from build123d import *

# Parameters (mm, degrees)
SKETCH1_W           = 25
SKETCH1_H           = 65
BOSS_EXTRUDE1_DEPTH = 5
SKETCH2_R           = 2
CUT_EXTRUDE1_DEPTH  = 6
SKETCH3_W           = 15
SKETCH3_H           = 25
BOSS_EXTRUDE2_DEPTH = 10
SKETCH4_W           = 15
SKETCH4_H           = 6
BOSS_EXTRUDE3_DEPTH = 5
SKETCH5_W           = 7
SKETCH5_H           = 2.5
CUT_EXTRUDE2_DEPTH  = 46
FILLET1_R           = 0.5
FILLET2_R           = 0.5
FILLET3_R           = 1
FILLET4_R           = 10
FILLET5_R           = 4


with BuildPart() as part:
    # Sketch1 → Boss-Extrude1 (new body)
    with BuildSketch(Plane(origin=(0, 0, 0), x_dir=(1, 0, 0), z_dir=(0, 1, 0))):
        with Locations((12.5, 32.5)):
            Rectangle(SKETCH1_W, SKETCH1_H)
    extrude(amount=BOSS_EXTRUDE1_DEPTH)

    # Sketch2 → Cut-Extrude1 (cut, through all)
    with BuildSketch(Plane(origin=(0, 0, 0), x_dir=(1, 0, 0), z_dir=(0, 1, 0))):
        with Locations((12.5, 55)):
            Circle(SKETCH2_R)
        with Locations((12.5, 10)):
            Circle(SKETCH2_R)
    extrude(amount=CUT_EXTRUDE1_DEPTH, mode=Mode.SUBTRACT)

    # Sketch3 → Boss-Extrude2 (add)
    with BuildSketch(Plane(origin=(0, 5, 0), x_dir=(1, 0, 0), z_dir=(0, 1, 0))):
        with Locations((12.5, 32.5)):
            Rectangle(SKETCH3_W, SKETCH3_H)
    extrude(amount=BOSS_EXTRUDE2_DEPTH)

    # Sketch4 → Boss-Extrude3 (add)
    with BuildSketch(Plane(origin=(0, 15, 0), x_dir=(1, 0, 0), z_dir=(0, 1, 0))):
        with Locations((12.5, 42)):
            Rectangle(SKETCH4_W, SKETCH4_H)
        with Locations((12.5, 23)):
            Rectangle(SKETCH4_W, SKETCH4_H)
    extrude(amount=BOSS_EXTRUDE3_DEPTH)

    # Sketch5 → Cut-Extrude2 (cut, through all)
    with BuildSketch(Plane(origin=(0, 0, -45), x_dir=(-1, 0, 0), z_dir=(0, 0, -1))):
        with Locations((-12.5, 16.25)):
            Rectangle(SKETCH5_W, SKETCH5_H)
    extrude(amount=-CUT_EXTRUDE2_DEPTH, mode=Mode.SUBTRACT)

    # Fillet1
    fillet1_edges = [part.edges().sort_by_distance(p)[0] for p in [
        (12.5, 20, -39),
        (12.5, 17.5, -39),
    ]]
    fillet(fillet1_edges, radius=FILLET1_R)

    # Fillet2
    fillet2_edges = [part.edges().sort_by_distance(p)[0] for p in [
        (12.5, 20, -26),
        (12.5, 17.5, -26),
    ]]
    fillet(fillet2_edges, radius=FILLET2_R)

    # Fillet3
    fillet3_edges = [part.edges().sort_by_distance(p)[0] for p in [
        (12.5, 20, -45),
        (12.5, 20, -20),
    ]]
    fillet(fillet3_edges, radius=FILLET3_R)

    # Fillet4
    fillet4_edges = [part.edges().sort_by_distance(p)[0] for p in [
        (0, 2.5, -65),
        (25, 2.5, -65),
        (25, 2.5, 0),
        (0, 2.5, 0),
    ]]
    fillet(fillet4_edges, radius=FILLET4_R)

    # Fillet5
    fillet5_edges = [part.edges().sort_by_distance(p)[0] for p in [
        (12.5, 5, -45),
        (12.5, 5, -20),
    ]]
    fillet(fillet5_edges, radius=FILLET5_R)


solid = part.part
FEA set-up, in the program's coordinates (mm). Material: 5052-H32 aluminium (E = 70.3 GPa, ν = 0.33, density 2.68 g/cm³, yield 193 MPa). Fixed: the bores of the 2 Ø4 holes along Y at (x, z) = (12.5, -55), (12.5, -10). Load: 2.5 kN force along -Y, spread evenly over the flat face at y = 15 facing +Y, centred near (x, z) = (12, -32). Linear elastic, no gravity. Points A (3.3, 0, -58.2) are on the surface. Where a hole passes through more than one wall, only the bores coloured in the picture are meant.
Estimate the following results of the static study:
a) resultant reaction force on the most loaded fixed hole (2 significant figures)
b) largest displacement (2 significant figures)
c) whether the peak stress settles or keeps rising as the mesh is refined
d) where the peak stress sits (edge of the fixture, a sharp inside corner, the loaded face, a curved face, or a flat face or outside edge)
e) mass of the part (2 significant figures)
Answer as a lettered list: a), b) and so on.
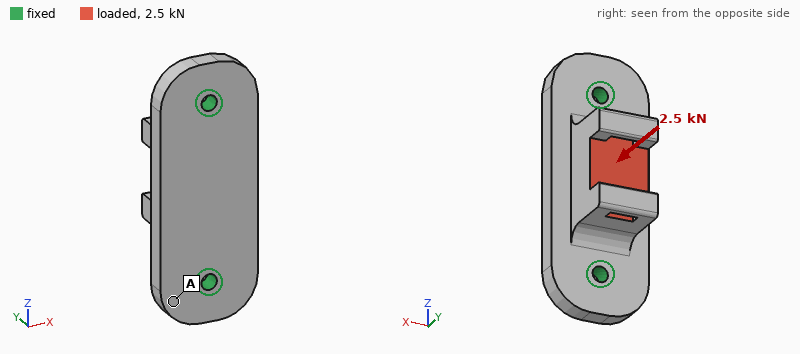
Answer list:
a) 1.4 kN
b) 23 µm
c) keeps rising
d) edge of the fixture
e) 32 g
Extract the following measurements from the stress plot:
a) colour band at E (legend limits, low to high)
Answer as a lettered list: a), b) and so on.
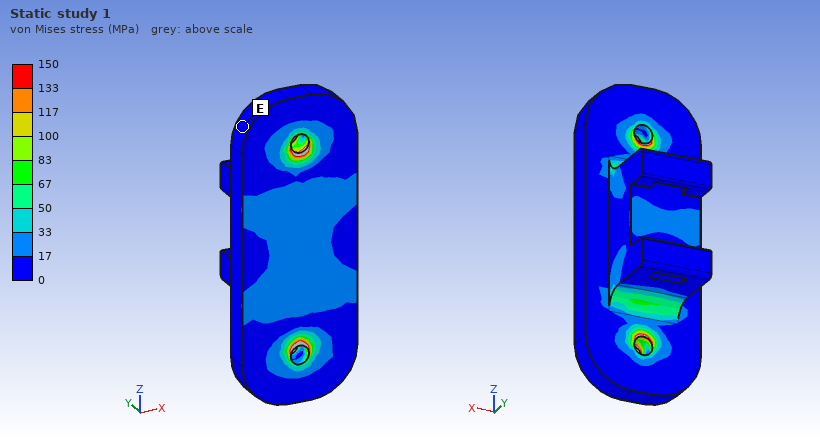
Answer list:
a) 0 to 17 MPa
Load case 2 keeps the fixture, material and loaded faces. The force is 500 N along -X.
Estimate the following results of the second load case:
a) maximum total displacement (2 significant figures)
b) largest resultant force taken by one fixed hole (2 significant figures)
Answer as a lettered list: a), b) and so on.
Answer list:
a) 27 µm
b) 250 N
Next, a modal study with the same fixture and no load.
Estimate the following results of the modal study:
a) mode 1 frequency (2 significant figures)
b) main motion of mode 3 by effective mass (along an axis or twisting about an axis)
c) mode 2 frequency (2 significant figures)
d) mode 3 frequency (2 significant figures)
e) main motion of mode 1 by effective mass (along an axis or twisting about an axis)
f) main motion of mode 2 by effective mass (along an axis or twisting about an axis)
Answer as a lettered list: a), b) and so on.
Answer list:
a) 7700 Hz
b) along X
c) 12 kHz
d) 19 kHz
e) along X
f) along Y
